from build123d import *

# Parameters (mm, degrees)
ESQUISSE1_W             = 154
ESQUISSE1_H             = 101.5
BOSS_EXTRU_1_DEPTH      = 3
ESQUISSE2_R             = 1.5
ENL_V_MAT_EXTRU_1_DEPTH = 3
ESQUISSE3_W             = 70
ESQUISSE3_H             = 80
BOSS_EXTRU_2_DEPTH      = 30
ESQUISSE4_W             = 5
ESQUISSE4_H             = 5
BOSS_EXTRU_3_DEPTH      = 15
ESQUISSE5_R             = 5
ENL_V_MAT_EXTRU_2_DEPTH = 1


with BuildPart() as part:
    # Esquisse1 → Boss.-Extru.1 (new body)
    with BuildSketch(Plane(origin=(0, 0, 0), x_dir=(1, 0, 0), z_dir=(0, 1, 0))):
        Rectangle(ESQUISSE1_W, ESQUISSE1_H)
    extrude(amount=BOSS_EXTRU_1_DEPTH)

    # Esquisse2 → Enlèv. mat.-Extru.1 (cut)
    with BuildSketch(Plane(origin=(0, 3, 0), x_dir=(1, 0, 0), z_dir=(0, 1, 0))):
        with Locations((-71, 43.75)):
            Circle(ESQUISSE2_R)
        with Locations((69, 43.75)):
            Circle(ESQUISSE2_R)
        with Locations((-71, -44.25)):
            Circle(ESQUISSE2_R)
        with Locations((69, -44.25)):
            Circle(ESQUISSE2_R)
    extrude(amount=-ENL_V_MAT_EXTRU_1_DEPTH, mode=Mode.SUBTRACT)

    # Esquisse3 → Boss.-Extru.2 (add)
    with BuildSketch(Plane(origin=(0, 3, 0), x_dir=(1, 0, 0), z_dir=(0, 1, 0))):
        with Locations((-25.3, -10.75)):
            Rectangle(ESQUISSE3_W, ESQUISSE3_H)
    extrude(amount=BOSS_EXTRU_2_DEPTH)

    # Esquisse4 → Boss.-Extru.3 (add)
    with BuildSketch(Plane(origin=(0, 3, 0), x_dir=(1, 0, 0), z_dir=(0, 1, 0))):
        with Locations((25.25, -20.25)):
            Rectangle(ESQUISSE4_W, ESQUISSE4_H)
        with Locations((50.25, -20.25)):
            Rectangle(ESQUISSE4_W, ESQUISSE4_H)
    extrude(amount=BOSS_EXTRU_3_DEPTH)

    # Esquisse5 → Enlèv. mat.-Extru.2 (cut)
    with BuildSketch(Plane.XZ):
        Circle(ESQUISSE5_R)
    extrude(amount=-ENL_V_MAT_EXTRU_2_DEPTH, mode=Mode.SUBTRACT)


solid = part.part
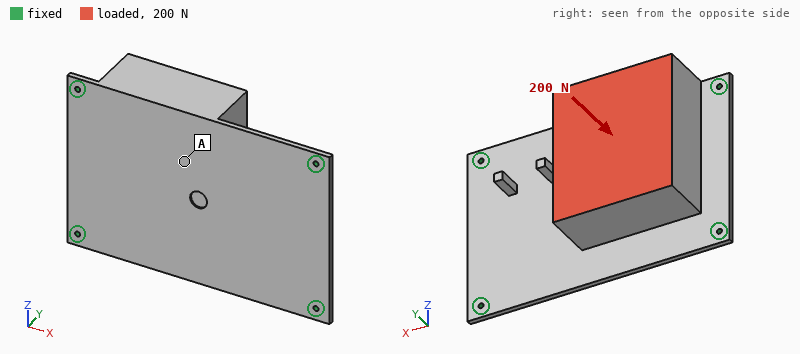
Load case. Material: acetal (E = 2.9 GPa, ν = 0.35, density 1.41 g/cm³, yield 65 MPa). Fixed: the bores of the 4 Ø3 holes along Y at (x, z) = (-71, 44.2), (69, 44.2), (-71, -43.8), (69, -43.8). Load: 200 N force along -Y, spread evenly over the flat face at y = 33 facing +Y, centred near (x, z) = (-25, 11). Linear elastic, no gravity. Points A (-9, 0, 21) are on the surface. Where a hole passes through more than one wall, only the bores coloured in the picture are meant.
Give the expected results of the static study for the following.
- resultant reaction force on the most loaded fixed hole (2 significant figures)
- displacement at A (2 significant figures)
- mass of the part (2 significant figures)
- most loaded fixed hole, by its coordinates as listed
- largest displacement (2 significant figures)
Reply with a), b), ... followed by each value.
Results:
a) 94 N
b) 1.5 mm
c) 300 g
d) (-71, 44.2)
e) 2.2 mm
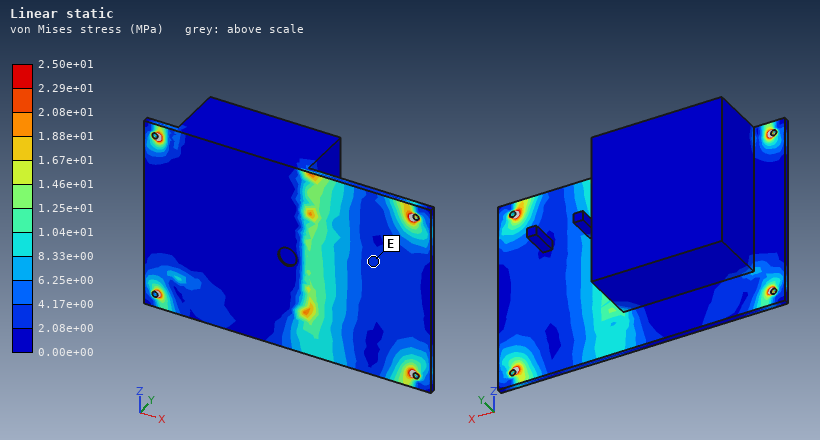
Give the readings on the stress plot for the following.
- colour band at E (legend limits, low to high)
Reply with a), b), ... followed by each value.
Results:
a) 2.08e+00 to 4.17e+00 MPa
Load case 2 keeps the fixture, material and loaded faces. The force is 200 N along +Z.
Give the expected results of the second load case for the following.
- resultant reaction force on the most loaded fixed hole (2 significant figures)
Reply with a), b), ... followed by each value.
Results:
a) 120 N
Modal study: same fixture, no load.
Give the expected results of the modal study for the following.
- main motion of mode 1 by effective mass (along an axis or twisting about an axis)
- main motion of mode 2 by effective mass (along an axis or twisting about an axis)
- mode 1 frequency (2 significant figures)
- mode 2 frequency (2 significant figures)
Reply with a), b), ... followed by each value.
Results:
a) along Y
b) along Z
c) 110 Hz
d) 290 Hz
